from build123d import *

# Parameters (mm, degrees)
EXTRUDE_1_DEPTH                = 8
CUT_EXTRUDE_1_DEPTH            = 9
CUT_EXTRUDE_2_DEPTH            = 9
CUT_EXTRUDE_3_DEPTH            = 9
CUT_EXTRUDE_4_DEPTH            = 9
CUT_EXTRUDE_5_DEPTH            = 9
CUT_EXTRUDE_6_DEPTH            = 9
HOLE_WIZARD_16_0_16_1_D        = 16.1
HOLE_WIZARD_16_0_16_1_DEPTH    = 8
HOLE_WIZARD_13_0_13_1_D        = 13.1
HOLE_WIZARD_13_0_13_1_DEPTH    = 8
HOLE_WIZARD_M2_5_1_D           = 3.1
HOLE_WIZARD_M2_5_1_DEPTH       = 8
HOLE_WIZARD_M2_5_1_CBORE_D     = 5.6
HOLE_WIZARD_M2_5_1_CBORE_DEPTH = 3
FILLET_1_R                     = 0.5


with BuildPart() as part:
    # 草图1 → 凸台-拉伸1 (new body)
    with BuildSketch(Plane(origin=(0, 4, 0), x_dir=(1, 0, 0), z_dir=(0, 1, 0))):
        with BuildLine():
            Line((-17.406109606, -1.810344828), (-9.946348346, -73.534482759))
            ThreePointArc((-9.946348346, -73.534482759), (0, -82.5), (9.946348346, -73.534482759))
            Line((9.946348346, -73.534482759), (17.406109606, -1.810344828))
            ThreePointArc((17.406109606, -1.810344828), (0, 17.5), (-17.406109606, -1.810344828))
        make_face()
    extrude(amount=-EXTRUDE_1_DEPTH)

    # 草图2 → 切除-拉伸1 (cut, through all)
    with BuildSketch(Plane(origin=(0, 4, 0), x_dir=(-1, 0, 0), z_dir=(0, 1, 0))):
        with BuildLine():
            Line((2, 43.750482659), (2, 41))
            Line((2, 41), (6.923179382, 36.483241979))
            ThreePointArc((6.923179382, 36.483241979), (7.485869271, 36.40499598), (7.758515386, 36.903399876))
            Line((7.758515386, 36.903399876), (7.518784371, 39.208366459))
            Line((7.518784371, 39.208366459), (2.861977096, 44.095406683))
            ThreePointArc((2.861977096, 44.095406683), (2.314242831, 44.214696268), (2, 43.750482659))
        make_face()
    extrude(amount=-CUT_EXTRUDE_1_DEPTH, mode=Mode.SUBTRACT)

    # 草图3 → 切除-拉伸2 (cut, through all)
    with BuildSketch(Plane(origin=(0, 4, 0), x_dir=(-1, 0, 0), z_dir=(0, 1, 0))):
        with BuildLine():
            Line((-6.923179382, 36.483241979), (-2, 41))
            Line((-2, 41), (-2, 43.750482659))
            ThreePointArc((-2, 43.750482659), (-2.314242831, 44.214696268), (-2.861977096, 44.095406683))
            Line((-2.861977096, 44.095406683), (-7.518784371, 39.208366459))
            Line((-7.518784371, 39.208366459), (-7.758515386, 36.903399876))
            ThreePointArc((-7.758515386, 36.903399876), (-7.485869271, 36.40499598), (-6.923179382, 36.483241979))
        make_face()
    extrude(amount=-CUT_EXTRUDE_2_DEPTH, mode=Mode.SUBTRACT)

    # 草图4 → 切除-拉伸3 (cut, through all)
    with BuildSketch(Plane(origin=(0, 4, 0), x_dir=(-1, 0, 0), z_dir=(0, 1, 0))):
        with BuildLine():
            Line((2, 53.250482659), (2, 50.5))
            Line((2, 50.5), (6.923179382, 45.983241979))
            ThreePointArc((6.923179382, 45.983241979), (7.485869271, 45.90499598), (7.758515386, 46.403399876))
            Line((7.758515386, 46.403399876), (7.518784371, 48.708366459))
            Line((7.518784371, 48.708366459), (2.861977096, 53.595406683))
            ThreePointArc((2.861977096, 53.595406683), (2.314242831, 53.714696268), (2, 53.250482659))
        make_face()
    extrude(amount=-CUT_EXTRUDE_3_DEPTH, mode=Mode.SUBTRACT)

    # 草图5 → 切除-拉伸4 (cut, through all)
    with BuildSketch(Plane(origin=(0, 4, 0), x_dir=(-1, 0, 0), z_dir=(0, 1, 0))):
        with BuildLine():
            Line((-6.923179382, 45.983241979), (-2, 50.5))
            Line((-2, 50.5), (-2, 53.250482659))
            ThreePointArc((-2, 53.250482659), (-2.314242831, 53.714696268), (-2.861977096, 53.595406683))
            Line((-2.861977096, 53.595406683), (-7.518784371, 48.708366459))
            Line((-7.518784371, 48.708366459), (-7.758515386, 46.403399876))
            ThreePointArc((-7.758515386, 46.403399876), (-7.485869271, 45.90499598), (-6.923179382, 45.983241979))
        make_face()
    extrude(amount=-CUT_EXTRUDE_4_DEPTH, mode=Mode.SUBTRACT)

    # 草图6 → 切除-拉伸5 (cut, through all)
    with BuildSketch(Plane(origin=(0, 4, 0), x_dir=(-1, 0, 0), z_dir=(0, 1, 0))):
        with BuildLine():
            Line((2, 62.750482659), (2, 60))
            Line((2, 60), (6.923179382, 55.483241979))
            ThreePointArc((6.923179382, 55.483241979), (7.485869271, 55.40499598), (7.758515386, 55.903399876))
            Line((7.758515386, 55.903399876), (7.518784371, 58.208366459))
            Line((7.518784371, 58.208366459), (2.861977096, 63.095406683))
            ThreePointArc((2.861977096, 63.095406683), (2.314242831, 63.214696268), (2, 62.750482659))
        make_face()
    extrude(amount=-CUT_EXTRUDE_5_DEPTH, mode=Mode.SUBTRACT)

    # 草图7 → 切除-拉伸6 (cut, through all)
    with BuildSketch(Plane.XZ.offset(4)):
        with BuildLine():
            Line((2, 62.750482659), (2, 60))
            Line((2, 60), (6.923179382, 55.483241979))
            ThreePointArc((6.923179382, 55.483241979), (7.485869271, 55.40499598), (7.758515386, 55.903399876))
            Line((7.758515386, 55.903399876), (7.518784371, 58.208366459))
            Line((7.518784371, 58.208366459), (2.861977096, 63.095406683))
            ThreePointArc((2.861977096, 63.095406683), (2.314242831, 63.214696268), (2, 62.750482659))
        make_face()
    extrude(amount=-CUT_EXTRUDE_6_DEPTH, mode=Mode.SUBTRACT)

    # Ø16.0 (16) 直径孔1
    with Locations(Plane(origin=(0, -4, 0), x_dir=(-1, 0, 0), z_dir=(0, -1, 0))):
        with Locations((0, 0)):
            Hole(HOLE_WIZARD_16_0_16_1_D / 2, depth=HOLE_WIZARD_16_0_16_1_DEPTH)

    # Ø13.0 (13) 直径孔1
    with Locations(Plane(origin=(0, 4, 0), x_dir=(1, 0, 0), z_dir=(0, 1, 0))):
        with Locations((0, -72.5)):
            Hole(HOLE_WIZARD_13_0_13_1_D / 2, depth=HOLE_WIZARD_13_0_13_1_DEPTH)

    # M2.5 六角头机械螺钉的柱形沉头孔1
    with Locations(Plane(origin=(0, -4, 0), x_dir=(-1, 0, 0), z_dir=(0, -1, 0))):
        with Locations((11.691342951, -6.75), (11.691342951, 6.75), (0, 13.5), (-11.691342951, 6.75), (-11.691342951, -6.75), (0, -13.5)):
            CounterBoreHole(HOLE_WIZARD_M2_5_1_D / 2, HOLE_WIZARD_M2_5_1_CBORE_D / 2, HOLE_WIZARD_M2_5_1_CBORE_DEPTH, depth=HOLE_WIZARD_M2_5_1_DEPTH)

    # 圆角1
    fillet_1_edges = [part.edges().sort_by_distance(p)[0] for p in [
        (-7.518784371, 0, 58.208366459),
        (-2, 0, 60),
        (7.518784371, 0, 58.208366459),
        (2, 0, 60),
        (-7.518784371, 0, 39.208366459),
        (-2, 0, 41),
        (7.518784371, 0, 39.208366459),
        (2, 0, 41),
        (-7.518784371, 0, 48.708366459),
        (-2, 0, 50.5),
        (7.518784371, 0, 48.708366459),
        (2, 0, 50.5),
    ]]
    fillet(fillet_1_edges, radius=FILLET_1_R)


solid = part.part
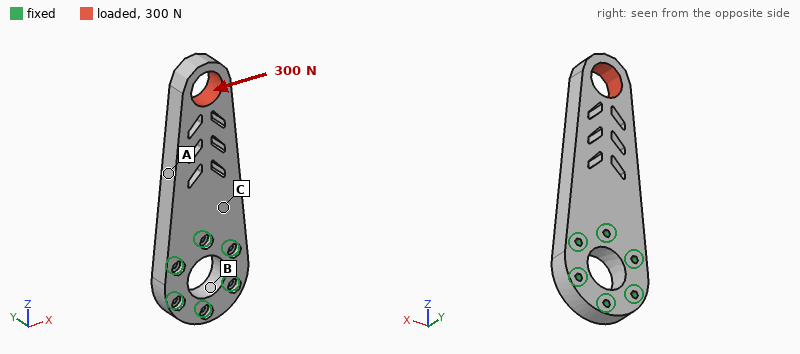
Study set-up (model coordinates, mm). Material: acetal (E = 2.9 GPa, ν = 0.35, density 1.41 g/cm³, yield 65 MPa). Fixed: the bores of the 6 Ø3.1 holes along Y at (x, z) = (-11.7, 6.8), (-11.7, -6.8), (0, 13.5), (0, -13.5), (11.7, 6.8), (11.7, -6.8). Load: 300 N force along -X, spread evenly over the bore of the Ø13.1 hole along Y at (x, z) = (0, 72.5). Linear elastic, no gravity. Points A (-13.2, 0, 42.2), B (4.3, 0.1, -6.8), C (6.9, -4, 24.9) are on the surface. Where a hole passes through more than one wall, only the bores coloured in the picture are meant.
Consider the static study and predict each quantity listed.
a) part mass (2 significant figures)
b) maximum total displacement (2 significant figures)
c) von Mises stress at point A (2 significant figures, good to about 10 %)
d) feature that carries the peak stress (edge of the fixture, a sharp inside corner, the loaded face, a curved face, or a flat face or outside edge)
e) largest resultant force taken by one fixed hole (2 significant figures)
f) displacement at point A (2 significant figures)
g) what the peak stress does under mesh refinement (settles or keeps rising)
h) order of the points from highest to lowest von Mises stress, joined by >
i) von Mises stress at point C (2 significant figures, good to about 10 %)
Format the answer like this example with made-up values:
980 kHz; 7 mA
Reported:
24 g; 1.0 mm; 11 MPa; edge of the fixture; 600 N; 0.29 mm; keeps rising; A > C > B; 4.6 MPa
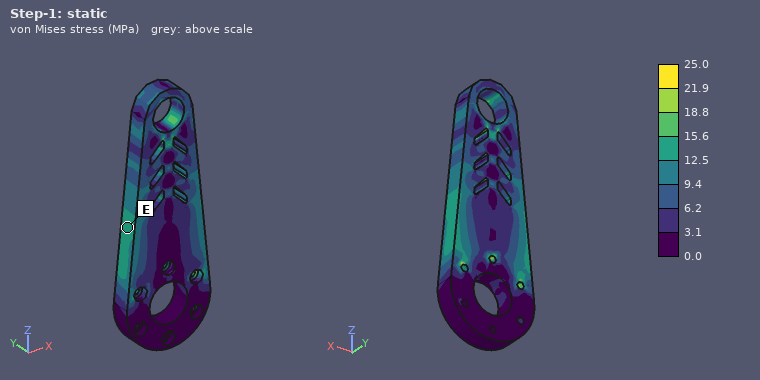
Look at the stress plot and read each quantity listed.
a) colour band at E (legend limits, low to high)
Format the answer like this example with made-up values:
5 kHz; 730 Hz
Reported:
12.5 to 15.6 MPa
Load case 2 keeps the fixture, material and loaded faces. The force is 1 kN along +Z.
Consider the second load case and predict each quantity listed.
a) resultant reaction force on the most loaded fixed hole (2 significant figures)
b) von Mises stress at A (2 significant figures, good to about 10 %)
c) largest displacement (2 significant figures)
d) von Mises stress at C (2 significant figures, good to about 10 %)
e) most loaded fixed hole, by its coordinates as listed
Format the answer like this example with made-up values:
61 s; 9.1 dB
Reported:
410 N; 7.7 MPa; 0.29 mm; 4.0 MPa; (0, 13.5)
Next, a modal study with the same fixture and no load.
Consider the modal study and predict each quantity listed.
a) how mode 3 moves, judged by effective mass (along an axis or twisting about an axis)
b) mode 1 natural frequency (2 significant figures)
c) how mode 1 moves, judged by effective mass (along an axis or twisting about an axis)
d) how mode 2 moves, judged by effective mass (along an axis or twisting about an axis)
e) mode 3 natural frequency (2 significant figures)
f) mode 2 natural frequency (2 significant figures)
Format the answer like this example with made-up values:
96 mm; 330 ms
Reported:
twisting about Z; 490 Hz; along Y; along X; 2000 Hz; 1500 Hz
